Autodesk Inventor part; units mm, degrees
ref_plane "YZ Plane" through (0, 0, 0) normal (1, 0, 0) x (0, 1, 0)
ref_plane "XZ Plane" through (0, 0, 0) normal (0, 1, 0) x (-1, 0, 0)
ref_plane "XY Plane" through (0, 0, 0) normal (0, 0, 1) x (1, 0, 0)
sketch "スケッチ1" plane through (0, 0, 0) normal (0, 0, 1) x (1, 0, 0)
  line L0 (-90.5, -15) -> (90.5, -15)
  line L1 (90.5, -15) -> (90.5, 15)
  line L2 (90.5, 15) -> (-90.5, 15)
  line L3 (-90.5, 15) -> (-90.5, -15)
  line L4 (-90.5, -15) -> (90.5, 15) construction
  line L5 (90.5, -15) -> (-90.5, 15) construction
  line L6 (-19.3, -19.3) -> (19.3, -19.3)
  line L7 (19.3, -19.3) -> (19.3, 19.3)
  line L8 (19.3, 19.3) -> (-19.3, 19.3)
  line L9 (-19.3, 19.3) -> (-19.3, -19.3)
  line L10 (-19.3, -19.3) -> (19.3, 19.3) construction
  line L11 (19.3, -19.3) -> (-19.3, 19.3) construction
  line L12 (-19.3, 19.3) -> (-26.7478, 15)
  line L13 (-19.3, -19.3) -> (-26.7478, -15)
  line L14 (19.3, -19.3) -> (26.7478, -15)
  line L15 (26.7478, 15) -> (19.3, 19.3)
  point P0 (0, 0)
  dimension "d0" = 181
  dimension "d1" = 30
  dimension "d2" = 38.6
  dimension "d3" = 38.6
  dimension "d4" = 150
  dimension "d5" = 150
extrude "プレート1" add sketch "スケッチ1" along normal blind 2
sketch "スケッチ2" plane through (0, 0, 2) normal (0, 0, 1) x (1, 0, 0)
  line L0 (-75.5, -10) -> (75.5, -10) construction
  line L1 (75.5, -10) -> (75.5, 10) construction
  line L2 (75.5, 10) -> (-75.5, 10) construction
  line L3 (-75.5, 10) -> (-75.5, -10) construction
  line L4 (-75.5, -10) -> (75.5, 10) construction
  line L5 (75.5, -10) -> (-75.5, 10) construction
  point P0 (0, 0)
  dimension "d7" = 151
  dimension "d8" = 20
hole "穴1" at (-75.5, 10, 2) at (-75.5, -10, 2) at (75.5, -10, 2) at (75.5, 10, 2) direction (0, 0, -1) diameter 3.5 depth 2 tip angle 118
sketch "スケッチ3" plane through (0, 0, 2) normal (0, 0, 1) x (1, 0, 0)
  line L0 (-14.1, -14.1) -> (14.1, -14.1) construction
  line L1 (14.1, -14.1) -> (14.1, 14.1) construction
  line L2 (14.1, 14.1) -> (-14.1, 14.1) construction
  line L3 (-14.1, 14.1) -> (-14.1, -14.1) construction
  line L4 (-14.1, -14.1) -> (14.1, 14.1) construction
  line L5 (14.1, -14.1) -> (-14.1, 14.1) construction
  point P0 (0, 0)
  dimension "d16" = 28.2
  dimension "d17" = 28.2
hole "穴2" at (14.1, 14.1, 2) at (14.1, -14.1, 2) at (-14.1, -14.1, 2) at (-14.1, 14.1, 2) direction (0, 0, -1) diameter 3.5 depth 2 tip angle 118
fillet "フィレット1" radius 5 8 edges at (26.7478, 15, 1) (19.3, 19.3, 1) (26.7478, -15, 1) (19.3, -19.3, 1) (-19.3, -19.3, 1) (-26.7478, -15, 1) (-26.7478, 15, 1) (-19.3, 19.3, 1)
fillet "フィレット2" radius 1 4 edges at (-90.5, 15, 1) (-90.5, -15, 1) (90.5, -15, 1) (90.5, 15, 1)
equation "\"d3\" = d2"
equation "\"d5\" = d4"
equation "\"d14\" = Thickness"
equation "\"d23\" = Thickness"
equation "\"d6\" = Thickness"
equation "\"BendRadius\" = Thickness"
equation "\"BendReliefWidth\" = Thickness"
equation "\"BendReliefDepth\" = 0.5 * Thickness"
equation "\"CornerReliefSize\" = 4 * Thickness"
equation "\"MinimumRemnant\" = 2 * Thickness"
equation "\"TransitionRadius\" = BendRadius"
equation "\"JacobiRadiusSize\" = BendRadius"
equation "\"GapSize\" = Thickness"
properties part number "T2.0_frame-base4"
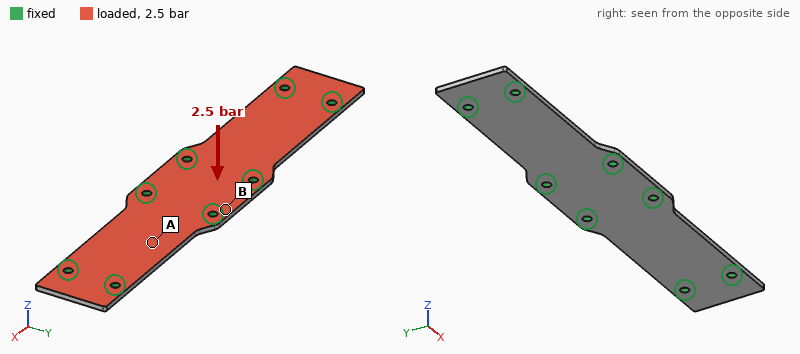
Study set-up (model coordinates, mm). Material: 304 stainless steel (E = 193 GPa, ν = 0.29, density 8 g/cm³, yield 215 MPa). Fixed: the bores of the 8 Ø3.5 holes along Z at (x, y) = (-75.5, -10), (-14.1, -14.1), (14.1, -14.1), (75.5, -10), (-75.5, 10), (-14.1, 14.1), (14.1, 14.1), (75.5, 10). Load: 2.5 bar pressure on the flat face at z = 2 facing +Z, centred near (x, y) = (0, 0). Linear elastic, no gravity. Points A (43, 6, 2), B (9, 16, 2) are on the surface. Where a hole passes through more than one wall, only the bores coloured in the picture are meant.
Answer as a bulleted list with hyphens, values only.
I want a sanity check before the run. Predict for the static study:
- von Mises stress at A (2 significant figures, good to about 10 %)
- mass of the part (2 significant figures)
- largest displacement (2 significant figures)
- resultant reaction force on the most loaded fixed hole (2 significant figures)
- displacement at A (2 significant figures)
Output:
- 50 MPa
- 92 g
- 69 µm
- 190 N
- 66 µm
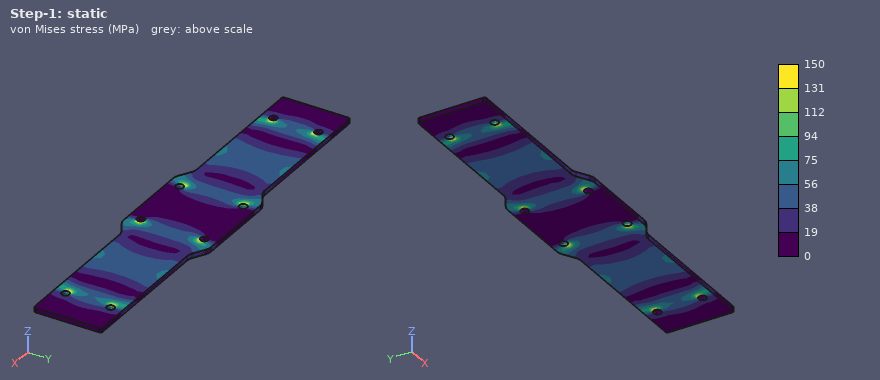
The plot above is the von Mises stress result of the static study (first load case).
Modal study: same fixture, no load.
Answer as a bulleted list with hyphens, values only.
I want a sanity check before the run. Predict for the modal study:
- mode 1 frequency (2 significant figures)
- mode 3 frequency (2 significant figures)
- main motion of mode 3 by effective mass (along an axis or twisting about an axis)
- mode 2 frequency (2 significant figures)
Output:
- 2800 Hz
- 4800 Hz
- twisting about X
- 2800 Hz
